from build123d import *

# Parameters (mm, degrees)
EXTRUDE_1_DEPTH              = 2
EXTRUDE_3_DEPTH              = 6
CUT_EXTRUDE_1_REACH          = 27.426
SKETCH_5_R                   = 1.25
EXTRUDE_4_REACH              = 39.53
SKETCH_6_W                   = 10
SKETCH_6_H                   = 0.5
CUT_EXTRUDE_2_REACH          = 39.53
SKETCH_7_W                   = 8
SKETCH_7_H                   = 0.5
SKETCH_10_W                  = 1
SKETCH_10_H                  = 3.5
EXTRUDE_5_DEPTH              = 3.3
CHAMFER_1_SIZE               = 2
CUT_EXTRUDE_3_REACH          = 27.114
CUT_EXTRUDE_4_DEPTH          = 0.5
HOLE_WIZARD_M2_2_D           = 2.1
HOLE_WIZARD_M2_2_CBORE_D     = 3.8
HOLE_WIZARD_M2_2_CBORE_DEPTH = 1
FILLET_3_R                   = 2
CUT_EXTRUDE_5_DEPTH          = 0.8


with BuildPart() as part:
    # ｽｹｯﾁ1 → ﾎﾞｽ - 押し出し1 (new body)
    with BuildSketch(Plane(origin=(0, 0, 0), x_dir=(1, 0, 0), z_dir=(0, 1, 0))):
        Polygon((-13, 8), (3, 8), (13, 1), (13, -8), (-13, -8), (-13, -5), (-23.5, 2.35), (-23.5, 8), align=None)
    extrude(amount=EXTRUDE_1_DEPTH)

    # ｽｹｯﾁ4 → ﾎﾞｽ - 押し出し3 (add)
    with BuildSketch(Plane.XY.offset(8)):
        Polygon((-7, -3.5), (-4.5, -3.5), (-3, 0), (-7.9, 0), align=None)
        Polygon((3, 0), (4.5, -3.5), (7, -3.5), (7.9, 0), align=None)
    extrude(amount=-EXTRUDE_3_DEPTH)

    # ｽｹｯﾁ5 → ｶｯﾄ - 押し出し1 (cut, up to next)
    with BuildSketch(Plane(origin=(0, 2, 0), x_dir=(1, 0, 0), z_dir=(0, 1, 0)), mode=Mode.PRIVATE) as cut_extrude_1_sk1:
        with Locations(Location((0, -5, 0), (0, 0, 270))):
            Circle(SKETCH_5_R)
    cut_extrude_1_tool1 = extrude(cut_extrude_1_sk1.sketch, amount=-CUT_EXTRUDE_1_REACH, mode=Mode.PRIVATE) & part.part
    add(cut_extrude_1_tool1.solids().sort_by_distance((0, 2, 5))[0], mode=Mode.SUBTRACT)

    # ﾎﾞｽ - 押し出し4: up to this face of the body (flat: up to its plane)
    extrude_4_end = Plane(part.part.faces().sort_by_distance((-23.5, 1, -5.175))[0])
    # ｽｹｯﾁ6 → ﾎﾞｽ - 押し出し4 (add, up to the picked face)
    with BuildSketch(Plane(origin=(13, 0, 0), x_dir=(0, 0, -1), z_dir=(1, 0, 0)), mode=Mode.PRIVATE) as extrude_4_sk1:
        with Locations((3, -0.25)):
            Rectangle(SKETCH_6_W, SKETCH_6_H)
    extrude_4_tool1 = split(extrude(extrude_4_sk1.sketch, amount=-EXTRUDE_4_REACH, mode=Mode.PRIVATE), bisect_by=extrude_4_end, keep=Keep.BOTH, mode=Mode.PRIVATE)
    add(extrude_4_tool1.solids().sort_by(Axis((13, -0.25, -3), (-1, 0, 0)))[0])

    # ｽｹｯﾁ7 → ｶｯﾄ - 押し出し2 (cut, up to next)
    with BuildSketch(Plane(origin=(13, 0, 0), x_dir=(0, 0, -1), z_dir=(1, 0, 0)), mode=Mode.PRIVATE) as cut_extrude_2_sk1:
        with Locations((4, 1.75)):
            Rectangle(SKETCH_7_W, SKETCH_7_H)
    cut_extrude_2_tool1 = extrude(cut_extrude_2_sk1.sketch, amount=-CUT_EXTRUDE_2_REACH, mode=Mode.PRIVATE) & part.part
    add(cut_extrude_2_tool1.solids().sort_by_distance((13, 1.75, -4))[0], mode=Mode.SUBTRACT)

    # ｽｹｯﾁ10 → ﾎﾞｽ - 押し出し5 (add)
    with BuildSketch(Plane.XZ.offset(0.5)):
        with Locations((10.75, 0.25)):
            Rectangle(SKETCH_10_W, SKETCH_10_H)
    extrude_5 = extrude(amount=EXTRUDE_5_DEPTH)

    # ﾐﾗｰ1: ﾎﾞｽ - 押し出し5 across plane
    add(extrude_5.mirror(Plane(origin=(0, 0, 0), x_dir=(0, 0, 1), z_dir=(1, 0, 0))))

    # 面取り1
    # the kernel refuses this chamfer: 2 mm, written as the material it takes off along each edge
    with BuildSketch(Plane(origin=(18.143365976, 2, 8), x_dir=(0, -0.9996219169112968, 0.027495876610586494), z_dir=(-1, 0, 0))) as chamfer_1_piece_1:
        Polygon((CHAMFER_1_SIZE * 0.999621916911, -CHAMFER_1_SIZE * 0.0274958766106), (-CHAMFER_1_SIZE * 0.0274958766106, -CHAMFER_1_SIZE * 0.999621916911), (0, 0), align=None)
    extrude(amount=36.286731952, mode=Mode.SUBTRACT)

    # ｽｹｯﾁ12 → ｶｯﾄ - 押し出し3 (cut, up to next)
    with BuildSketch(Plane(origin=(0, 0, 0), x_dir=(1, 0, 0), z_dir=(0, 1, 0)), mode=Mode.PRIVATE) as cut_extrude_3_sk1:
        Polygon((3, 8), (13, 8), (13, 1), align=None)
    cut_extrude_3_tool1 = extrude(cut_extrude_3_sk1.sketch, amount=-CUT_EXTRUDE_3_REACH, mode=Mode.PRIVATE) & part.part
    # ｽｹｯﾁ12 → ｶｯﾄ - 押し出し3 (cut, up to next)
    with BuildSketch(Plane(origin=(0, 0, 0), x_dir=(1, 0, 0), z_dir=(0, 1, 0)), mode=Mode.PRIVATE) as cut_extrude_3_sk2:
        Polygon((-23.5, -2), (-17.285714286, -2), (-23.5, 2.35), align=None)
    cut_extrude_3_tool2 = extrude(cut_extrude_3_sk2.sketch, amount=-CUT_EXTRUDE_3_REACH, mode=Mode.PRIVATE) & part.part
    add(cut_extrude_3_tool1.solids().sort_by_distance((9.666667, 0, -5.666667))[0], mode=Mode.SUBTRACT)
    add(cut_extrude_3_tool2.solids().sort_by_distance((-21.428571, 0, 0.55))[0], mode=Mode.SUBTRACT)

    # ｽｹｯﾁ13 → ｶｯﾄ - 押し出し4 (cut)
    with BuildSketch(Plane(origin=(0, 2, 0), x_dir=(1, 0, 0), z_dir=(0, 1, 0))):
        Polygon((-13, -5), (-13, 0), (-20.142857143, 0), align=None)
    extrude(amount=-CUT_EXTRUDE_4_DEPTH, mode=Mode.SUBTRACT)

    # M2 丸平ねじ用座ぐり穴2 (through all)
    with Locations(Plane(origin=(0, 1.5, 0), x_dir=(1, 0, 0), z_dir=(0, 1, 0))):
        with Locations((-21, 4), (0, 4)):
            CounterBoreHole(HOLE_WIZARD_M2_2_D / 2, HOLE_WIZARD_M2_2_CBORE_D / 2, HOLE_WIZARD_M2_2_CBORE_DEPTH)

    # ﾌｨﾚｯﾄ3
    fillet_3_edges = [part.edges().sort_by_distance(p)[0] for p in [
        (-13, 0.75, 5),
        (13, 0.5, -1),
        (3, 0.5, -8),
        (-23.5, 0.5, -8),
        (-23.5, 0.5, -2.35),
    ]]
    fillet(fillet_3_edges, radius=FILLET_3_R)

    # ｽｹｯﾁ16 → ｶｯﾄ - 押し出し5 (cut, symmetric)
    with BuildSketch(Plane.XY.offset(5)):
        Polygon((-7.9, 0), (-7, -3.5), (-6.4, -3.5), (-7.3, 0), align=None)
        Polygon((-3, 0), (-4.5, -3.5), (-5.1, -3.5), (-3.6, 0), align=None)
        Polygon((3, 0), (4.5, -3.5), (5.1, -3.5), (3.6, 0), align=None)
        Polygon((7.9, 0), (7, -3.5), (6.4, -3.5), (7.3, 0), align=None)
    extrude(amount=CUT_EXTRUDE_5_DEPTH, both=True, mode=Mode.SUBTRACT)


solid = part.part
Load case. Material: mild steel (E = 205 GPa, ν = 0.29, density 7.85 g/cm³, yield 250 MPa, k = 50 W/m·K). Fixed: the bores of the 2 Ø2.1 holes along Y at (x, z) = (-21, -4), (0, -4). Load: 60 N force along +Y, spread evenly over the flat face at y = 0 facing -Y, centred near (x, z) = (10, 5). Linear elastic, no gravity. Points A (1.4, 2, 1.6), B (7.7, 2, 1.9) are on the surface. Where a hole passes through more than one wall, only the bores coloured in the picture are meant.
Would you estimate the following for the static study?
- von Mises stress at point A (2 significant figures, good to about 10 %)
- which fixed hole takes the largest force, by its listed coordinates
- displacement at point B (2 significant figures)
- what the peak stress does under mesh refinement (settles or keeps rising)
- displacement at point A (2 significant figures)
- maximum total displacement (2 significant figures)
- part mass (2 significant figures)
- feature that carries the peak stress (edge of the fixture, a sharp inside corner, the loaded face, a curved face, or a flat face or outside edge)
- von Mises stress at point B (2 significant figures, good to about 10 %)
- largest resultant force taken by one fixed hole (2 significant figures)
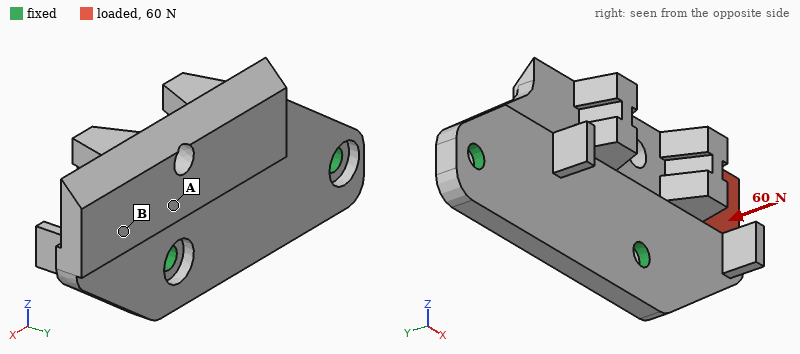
69 MPa
(0, -4)
25 µm
keeps rising
11 µm
54 µm
8.3 g
edge of the fixture
20 MPa
100 N
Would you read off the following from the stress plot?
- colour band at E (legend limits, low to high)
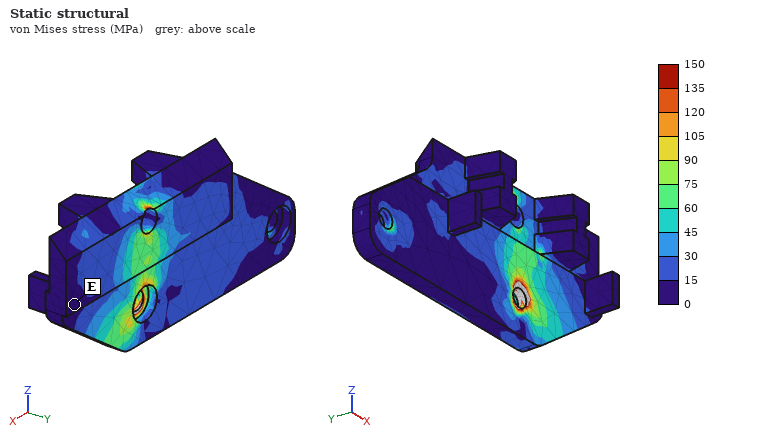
0 to 15 MPa
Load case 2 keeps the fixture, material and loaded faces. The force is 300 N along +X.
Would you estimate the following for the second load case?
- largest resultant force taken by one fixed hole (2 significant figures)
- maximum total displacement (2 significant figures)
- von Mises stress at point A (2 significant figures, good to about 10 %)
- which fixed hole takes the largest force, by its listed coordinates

220 N
19 µm
16 MPa
(0, -4)
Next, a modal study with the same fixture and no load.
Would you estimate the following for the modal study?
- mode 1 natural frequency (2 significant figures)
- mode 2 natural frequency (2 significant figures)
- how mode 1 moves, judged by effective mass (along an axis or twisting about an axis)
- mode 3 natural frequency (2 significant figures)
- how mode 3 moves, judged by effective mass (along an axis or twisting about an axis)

5300 Hz
7900 Hz
along Y
18 kHz
along Y
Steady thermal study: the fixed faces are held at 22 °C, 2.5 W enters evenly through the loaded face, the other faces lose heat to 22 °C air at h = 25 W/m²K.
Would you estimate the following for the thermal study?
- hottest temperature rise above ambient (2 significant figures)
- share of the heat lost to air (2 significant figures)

36 K
12 %
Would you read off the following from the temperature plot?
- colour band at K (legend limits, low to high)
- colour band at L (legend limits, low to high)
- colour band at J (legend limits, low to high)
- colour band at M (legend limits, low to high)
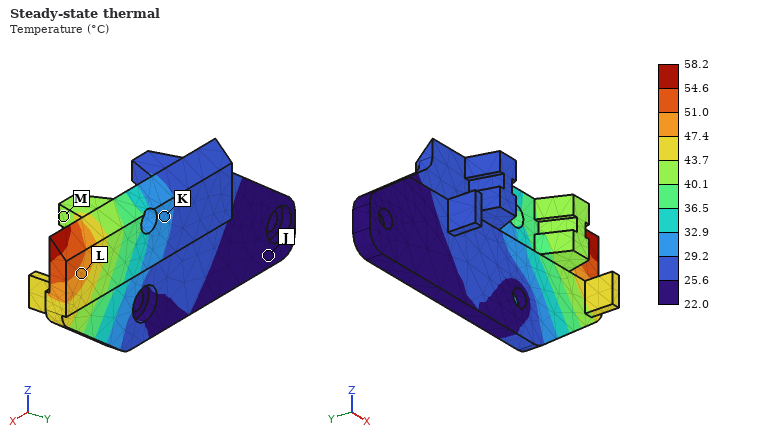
29.2 to 32.9 °C
47.4 to 51.0 °C
22.0 to 25.6 °C
40.1 to 43.7 °C
